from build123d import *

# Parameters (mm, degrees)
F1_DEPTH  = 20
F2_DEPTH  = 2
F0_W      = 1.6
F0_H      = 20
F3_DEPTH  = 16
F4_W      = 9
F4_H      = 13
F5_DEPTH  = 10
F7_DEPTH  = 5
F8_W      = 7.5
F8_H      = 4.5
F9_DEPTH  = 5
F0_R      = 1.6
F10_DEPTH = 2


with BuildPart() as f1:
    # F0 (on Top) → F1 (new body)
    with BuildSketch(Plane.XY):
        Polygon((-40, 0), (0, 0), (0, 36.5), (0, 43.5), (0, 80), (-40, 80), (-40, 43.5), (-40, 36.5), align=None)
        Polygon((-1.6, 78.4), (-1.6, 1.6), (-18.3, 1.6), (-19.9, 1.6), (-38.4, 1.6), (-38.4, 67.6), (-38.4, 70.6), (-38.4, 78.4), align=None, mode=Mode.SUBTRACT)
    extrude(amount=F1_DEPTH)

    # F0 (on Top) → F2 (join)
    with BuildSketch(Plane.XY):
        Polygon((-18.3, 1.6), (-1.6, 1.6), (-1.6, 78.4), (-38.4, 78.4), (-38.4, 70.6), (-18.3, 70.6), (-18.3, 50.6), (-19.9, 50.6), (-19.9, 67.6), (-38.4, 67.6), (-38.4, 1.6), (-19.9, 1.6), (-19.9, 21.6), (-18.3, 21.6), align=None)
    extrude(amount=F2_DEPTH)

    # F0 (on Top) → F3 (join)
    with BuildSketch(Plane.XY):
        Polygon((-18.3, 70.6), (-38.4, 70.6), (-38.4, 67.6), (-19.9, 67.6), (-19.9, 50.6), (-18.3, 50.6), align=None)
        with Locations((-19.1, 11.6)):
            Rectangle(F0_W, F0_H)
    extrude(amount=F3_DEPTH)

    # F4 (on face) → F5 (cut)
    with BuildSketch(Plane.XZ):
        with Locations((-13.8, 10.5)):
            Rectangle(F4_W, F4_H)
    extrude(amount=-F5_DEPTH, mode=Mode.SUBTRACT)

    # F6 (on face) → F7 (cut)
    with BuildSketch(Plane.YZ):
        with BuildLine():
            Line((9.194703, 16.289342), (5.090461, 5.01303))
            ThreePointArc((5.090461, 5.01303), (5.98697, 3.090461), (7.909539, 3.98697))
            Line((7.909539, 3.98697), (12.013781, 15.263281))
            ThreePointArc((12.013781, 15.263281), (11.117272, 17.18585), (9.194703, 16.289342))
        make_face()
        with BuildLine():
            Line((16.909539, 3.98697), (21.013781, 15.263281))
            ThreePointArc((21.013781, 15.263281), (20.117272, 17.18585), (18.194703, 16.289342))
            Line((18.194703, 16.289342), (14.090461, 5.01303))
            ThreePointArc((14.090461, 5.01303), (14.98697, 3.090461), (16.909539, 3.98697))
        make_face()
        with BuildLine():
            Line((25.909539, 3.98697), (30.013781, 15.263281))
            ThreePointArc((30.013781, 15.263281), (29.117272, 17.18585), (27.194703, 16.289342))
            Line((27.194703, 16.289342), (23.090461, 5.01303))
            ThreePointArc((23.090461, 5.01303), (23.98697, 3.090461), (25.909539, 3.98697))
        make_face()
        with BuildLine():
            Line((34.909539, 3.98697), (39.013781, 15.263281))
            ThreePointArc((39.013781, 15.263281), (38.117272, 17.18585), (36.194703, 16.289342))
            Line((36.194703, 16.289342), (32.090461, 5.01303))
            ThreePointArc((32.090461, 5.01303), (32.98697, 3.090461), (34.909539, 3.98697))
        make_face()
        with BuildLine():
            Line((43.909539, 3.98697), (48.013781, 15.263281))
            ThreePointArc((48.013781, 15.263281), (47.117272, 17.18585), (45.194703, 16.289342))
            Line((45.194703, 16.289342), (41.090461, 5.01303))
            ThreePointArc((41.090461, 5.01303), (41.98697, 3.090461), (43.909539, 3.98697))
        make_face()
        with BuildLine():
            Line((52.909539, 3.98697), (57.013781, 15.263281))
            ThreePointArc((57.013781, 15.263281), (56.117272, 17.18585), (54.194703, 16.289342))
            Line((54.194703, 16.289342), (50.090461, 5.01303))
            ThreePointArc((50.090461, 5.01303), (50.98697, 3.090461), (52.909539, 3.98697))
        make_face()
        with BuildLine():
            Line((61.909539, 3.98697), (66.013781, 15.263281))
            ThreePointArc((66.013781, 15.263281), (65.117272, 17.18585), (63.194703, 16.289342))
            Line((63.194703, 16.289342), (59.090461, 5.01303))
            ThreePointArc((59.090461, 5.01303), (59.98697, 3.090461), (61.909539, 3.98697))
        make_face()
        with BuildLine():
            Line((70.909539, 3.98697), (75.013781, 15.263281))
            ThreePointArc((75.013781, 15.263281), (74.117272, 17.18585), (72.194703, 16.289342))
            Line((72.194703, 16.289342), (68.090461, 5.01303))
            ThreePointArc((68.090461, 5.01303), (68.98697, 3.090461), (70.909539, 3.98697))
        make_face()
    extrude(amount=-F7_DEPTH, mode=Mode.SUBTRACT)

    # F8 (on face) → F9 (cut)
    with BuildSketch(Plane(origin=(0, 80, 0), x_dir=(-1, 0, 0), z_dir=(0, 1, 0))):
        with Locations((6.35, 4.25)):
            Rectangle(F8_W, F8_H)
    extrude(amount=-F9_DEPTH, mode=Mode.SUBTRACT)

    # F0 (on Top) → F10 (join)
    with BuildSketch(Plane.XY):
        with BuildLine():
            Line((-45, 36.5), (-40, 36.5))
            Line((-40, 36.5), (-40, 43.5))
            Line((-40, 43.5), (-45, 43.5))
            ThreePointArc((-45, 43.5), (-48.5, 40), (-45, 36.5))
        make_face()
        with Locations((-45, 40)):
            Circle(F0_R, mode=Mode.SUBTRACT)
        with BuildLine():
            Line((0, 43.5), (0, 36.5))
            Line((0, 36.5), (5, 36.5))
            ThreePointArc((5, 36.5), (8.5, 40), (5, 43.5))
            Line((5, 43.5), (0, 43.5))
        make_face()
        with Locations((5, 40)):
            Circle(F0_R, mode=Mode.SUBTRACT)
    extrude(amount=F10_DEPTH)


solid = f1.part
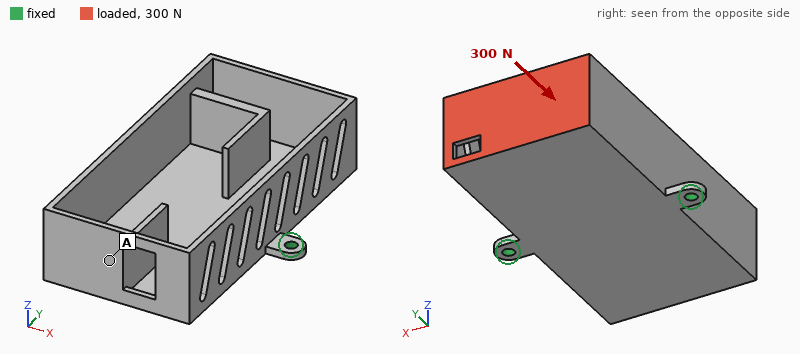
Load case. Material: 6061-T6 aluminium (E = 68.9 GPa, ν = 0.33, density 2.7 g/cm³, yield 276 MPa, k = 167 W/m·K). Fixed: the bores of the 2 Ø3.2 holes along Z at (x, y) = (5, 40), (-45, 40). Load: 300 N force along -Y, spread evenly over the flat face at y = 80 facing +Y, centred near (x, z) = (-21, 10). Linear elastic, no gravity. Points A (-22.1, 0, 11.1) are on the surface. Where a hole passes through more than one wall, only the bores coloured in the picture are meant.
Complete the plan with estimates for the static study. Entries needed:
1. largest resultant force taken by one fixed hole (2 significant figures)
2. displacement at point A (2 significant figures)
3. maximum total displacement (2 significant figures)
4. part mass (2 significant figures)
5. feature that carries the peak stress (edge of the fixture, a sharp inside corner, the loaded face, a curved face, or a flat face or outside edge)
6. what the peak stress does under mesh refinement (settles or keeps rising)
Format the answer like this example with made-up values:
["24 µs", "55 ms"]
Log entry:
["160 N", "0.49 mm", "0.59 mm", "38 g", "edge of the fixture", "keeps rising"]
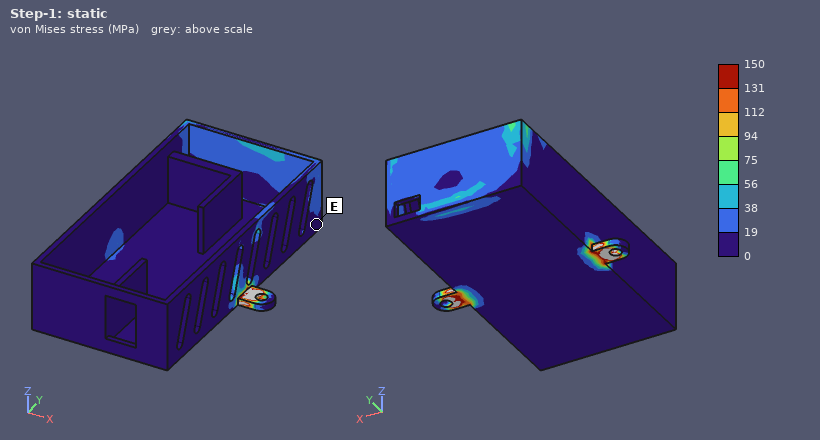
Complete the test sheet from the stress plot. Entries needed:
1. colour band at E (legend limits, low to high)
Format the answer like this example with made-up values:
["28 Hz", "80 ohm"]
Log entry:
["0 to 19 MPa"]
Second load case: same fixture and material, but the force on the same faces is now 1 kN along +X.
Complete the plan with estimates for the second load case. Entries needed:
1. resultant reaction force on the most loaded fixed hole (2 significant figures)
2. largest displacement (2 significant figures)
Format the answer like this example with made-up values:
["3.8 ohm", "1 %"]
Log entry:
["1.0 kN", "0.69 mm"]
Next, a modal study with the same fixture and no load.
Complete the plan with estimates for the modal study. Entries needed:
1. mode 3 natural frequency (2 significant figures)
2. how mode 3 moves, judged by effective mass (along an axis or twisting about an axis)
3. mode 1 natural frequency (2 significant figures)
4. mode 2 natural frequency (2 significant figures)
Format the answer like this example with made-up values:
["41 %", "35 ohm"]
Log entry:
["2500 Hz", "along Z", "450 Hz", "1500 Hz"]
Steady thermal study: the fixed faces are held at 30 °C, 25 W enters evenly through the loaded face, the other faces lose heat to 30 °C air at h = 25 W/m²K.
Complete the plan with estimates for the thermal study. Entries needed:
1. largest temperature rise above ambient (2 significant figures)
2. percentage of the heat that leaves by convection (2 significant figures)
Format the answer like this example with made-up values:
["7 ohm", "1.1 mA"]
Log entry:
["70 K", "44 %"]
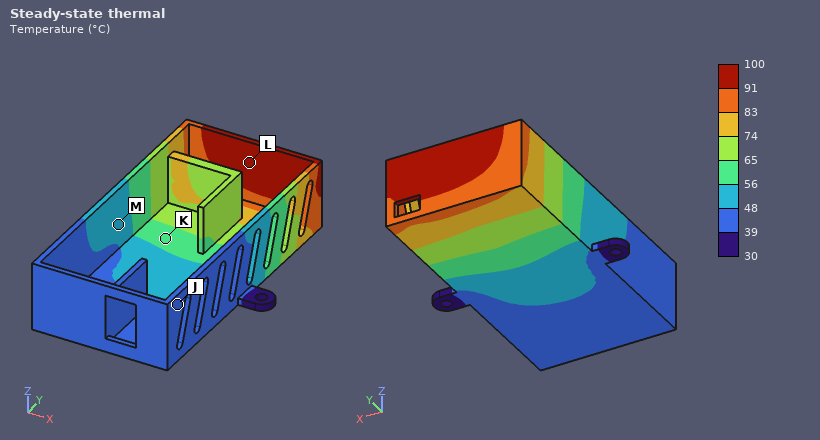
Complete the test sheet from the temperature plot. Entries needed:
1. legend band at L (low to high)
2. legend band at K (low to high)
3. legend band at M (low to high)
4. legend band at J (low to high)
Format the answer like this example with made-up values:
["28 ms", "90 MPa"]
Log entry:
["91 to 100 °C", "56 to 65 °C", "48 to 56 °C", "39 to 48 °C"]
